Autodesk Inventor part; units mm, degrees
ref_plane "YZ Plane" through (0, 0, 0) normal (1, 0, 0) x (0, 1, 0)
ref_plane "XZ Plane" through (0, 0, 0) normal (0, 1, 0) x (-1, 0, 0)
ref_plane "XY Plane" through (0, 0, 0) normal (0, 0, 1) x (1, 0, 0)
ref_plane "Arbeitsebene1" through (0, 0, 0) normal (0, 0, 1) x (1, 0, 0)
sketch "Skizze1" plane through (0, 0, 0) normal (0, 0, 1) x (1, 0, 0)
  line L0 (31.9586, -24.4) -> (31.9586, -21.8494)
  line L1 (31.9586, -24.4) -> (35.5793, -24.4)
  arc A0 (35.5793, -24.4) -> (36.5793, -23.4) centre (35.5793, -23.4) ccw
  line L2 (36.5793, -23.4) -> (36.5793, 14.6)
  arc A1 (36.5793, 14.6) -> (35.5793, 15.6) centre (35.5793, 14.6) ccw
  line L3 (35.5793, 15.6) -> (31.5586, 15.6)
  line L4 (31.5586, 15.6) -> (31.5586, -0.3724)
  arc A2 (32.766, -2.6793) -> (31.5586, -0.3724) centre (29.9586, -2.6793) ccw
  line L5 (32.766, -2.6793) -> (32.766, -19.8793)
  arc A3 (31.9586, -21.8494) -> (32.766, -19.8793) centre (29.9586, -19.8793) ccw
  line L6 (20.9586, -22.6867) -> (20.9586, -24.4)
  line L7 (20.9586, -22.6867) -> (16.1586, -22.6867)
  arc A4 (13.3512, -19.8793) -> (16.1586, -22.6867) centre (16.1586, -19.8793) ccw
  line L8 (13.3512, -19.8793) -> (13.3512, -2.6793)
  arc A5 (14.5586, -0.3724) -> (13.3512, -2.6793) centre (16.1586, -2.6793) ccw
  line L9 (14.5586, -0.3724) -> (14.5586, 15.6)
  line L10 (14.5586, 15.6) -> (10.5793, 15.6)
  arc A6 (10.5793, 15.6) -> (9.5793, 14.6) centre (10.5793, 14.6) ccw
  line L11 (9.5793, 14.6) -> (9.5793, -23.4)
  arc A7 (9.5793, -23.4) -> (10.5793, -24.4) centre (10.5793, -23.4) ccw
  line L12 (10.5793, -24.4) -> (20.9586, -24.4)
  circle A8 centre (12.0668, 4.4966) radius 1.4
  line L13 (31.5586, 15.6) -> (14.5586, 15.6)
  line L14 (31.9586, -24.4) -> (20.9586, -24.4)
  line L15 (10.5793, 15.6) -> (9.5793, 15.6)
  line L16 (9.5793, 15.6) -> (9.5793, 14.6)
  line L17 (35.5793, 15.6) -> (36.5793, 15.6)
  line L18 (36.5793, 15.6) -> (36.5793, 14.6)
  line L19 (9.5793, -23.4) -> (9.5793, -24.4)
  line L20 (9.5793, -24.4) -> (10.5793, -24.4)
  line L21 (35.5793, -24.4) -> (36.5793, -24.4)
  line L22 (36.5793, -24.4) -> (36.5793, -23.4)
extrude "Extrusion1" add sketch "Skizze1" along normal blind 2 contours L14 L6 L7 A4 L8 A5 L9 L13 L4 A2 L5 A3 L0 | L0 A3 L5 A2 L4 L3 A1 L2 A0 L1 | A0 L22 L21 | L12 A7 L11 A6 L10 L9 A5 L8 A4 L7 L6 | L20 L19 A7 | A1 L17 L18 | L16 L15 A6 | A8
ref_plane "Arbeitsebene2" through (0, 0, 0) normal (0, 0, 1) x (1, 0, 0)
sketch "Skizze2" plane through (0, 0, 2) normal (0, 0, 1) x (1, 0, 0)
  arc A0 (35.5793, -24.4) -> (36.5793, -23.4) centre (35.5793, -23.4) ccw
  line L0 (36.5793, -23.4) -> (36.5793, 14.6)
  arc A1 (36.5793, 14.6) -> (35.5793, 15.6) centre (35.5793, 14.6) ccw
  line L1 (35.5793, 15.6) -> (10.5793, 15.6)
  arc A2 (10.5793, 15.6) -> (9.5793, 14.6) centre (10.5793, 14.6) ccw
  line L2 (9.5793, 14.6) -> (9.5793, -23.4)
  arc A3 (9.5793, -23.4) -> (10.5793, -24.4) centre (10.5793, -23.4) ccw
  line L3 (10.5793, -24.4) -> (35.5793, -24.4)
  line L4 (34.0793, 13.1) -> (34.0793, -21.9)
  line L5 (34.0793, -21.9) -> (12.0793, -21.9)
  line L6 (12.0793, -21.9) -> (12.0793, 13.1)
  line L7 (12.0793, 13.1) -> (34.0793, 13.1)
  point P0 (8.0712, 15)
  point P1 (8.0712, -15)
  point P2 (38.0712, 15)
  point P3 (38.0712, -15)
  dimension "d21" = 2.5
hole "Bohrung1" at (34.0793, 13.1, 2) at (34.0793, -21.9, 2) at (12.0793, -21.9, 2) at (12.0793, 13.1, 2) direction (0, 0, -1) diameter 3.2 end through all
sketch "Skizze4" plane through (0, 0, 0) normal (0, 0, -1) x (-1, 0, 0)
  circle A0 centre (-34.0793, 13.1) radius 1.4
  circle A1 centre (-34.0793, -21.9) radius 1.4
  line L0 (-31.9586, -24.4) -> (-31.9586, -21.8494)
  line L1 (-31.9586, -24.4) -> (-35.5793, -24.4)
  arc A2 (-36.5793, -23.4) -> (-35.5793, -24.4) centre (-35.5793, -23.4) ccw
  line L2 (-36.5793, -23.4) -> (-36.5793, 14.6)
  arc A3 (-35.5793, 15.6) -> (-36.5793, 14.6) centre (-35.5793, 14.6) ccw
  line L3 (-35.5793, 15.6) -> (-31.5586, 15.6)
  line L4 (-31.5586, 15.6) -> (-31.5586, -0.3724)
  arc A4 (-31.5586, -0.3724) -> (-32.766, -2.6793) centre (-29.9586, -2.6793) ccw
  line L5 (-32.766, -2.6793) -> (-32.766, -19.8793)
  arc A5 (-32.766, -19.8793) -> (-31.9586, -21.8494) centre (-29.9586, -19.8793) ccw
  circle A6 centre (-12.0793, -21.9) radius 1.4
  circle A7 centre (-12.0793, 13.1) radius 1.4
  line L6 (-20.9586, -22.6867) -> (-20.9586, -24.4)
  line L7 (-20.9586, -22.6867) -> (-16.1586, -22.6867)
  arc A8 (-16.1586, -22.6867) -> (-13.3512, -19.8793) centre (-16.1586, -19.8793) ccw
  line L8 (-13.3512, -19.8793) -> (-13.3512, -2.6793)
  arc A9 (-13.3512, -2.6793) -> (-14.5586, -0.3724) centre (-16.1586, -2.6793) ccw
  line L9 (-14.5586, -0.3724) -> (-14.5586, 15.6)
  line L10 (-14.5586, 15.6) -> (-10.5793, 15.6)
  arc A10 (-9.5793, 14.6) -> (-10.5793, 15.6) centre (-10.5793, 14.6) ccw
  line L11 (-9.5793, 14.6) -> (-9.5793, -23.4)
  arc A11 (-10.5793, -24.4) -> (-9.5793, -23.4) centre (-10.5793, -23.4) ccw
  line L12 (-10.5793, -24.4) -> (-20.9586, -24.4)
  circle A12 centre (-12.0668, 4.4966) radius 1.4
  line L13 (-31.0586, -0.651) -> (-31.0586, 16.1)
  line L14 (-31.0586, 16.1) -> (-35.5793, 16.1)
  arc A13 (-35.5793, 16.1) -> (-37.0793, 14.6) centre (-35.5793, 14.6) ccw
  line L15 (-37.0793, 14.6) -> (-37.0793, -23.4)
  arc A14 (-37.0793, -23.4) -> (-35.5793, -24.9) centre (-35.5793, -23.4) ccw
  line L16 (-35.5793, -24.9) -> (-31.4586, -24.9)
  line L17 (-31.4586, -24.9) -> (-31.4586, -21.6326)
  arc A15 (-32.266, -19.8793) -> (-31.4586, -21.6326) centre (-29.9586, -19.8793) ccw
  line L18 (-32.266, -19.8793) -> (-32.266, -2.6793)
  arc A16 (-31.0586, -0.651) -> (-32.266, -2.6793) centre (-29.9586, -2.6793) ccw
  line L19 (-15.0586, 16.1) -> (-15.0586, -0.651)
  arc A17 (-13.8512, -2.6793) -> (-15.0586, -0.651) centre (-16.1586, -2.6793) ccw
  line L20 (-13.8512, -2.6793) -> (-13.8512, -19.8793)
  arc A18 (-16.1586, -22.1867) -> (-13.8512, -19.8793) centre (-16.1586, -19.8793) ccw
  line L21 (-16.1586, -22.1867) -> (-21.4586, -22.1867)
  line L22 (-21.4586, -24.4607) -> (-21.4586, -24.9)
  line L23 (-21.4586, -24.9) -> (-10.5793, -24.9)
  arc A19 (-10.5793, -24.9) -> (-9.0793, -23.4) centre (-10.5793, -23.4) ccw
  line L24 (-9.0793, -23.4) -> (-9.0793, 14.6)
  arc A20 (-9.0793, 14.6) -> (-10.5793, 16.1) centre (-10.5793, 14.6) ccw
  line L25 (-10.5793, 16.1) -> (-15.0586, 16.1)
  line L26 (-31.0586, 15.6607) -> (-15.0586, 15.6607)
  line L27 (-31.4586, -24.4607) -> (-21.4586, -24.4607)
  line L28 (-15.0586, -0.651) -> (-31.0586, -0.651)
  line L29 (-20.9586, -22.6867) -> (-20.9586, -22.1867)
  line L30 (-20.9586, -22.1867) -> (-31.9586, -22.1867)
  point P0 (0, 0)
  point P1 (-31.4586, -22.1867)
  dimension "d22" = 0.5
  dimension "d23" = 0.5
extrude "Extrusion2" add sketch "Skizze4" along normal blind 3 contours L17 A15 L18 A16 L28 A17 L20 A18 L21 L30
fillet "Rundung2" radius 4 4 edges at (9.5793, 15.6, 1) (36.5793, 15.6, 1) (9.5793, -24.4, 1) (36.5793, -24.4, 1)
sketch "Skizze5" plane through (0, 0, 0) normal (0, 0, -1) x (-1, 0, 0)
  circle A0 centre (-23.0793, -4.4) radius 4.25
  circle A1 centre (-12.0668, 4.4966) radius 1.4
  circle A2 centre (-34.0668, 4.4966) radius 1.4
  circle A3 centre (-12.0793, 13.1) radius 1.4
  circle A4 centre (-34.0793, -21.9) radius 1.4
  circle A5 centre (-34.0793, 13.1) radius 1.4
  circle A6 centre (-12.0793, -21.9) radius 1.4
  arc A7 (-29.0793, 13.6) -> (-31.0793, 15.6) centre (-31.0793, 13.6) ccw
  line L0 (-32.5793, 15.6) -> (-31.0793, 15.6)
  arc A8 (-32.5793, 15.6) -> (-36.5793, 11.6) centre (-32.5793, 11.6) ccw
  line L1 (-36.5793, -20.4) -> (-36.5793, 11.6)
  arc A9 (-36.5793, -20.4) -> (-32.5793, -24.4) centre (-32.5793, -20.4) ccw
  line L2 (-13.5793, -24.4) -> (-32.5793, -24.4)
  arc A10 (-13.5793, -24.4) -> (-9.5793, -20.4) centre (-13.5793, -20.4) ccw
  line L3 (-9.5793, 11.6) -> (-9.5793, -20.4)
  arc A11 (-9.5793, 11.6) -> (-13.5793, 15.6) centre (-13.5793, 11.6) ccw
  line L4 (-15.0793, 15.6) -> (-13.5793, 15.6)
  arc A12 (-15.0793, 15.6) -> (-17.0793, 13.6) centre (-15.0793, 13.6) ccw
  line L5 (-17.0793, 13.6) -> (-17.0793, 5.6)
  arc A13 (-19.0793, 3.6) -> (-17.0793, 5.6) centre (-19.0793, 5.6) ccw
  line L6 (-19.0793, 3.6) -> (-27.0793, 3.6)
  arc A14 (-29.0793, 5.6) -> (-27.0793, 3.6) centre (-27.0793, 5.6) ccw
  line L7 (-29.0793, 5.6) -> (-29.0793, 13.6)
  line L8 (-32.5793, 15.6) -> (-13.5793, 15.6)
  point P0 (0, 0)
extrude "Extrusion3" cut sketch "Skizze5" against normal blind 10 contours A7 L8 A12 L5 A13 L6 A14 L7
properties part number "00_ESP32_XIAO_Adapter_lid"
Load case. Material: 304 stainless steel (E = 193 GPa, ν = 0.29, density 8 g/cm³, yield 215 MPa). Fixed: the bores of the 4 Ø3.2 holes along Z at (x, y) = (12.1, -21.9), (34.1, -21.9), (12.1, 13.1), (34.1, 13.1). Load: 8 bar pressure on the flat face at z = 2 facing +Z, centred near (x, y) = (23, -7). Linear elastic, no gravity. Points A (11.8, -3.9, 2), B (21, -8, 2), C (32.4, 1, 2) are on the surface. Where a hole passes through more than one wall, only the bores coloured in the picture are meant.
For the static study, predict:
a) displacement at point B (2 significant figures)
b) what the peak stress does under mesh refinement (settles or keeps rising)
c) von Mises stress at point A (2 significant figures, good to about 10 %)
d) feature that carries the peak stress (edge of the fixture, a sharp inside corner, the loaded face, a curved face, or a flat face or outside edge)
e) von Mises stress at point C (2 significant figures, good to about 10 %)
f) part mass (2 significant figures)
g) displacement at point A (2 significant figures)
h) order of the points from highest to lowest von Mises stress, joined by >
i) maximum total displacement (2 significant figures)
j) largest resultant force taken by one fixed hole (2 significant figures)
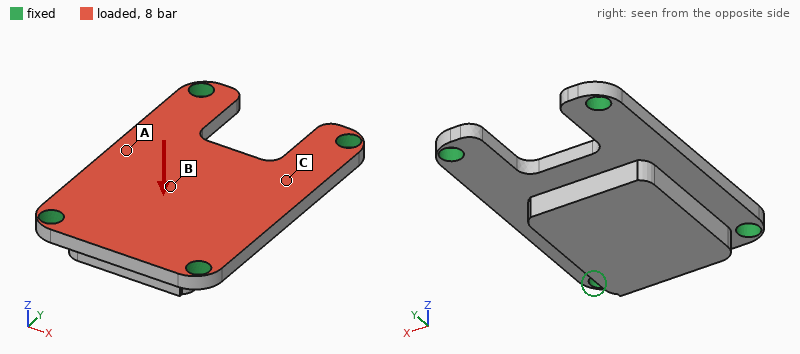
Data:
13 µm
keeps rising
36 MPa
edge of the fixture
62 MPa
24 g
17 µm
C > A > B
20 µm
220 N
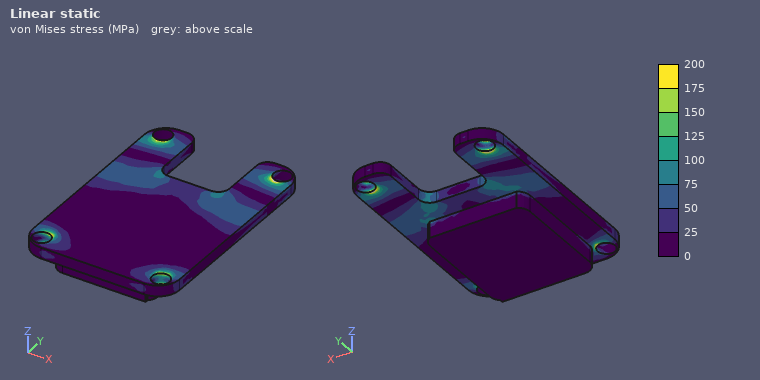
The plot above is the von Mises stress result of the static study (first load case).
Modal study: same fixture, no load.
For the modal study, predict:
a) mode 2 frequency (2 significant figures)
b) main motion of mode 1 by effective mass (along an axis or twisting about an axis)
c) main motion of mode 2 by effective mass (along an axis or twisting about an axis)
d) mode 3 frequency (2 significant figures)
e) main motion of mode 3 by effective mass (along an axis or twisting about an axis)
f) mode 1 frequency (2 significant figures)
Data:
15 kHz
along Z
twisting about Y
26 kHz
along X
7300 Hz
